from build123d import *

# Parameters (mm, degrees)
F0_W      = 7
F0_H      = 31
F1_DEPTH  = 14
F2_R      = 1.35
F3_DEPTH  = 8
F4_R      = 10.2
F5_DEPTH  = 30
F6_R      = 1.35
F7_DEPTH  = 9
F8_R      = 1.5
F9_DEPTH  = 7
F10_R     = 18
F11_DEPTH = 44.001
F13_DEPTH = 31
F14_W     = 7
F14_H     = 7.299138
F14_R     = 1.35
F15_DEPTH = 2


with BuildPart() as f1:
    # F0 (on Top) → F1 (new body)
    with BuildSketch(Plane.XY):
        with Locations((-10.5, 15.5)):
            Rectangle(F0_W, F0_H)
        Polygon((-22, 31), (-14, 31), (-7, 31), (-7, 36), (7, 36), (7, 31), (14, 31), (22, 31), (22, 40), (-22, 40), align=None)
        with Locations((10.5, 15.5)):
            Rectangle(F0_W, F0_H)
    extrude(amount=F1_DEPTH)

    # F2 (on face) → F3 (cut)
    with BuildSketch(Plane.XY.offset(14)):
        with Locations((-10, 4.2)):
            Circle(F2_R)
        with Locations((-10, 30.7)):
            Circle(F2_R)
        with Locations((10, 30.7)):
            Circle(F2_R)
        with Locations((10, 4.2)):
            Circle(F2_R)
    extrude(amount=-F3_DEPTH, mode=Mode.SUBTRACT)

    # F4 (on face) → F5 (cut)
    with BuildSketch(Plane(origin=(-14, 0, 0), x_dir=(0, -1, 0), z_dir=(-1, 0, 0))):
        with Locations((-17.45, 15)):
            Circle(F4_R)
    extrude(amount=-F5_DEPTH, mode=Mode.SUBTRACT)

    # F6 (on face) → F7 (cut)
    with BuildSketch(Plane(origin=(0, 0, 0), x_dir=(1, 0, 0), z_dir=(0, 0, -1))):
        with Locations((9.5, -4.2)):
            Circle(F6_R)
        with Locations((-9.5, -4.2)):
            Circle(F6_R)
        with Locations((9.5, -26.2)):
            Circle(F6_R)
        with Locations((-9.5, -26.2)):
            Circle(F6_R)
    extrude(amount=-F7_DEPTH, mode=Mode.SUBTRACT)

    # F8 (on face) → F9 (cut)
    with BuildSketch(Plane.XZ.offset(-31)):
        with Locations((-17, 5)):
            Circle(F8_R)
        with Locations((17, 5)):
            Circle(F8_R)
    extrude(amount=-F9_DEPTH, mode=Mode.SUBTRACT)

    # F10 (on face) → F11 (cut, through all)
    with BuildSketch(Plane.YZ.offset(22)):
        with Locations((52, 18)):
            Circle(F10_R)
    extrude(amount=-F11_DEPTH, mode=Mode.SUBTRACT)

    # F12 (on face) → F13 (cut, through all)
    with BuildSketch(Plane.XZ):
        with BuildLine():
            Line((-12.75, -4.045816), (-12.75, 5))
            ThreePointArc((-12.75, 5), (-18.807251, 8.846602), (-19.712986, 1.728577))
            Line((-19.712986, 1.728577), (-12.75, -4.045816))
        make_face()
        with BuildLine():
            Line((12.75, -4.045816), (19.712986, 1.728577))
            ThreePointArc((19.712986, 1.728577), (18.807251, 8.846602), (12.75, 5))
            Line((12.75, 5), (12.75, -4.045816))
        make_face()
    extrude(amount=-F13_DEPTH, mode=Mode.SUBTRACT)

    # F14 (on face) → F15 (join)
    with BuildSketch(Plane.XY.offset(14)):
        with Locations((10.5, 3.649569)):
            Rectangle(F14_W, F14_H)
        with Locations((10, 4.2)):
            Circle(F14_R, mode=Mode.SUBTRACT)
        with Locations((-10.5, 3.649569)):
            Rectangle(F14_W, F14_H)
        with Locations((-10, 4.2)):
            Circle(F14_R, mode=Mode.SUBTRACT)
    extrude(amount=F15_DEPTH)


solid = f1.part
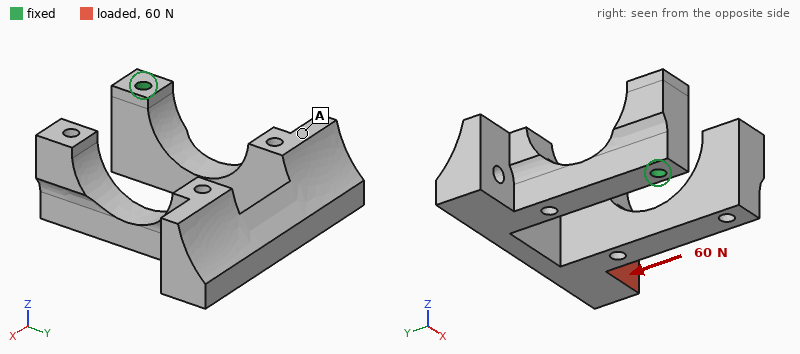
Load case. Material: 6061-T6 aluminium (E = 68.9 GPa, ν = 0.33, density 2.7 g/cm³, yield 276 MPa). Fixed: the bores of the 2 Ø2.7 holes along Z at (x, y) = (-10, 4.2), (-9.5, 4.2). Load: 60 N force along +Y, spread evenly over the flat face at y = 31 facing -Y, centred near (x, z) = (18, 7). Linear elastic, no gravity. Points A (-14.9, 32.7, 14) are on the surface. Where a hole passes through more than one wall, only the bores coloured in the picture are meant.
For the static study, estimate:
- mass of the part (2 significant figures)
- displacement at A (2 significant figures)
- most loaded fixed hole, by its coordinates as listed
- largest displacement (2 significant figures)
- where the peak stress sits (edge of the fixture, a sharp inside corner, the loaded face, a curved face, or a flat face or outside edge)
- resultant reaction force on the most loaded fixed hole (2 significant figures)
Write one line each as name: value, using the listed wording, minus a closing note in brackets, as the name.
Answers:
mass of the part: 18 g
displacement at A: 0.099 mm
most loaded fixed hole, by its coordinates as listed: (-9.5, 4.2)
largest displacement: 0.56 mm
where the peak stress sits: a curved face
resultant reaction force on the most loaded fixed hole: 90 N
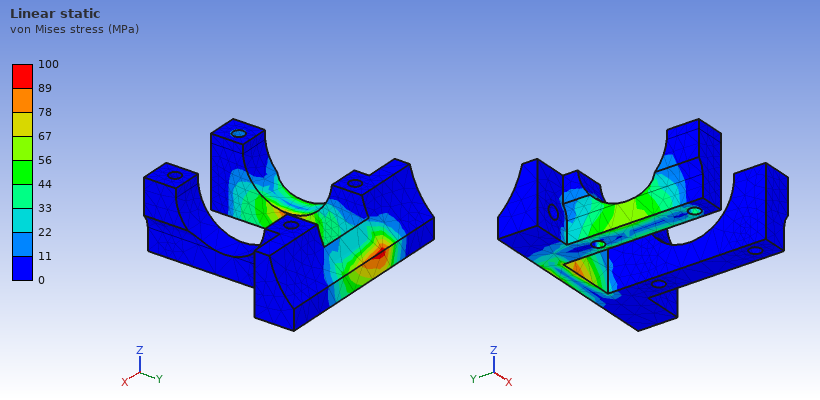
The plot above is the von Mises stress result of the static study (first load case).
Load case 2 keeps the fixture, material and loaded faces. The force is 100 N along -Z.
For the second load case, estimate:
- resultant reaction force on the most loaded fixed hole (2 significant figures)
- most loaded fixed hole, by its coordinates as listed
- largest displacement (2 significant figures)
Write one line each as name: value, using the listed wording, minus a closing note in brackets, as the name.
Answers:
resultant reaction force on the most loaded fixed hole: 140 N
most loaded fixed hole, by its coordinates as listed: (-9.5, 4.2)
largest displacement: 0.73 mm
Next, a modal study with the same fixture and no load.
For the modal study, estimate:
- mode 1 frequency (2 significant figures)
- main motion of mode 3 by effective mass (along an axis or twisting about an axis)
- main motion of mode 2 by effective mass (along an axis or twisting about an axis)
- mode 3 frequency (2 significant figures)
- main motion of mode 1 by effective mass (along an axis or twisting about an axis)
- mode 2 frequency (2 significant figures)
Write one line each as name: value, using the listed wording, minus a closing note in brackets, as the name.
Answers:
mode 1 frequency: 670 Hz
main motion of mode 3 by effective mass: along X
main motion of mode 2 by effective mass: along Z
mode 3 frequency: 1100 Hz
main motion of mode 1 by effective mass: along Y
mode 2 frequency: 740 Hz
